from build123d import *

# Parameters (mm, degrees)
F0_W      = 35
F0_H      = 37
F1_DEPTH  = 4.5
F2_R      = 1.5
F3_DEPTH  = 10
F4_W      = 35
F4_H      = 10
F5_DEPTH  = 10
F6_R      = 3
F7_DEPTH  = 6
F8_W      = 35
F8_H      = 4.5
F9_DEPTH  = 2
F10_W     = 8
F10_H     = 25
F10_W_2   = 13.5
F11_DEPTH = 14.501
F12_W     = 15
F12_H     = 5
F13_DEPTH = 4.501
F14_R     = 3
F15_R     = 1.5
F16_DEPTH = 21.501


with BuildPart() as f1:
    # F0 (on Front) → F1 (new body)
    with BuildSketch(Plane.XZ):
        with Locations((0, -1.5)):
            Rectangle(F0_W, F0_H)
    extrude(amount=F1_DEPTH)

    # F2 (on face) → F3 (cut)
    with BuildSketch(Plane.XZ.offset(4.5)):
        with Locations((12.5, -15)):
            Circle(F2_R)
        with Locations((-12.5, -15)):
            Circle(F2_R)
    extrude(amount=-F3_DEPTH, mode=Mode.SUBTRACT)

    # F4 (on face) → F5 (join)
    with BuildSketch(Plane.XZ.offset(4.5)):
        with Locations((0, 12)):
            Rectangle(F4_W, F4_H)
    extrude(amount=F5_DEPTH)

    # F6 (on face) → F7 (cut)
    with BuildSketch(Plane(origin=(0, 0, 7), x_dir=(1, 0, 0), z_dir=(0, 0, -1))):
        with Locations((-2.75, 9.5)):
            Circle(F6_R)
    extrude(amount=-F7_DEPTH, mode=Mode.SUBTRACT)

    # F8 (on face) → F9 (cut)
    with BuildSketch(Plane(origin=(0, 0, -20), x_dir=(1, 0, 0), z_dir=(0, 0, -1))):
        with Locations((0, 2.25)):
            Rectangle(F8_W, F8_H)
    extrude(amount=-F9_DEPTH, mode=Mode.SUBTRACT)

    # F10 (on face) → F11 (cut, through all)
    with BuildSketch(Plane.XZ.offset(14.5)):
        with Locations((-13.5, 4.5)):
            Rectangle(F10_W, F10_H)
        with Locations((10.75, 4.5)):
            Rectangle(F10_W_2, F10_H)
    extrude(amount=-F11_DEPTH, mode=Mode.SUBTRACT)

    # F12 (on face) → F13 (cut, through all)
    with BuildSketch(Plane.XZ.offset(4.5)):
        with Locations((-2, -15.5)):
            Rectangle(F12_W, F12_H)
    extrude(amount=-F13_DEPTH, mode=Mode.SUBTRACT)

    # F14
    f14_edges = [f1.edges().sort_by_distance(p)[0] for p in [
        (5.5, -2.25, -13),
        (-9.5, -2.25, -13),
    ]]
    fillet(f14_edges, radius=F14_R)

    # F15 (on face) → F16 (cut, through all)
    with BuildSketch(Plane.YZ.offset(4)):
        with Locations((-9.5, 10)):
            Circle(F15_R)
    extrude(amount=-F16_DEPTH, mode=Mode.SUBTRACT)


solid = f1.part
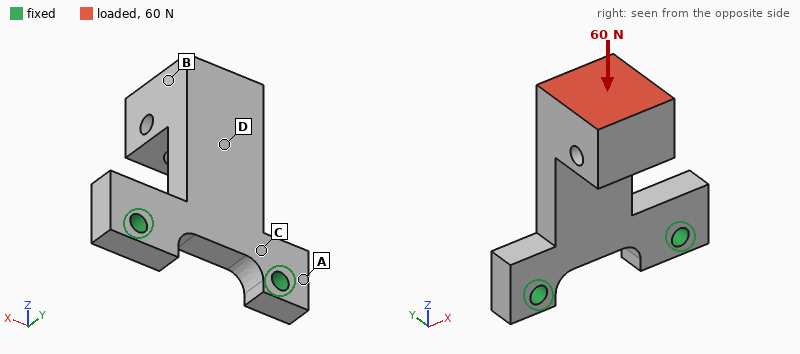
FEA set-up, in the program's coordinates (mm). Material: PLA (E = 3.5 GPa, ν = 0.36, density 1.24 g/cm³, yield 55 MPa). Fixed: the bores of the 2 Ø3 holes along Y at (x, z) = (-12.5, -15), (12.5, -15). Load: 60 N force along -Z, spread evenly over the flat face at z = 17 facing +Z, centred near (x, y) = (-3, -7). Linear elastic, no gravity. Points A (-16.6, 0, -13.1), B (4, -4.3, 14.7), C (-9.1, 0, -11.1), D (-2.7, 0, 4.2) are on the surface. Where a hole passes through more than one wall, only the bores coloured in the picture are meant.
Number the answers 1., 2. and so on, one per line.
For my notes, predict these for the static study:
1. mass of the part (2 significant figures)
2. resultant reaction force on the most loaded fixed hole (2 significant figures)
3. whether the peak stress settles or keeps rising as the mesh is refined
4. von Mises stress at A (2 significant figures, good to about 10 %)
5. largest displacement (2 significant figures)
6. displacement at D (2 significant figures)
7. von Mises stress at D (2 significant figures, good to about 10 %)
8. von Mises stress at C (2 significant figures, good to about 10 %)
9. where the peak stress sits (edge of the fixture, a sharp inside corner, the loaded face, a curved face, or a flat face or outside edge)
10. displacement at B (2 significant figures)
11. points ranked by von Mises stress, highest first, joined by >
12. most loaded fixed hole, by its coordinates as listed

1. 4.8 g
2. 42 N
3. keeps rising
4. 2.0 MPa
5. 0.58 mm
6. 0.21 mm
7. 5.2 MPa
8. 8.0 MPa
9. edge of the fixture
10. 0.45 mm
11. C > D > A > B
12. (-12.5, -15)
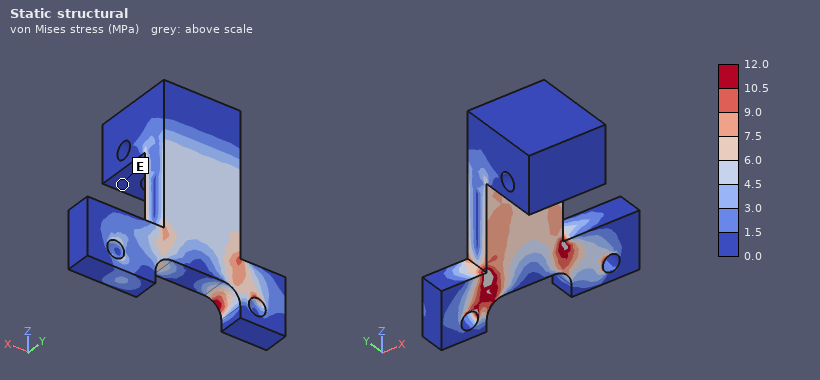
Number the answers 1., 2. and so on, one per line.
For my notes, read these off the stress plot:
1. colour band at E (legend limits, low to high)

1. 0.0 to 1.5 MPa
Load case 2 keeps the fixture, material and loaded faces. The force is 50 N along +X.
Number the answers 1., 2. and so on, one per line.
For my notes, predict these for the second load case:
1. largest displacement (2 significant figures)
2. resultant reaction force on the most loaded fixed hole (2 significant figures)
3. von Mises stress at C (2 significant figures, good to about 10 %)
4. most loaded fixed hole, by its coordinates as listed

1. 0.32 mm
2. 91 N
3. 7.9 MPa
4. (12.5, -15)
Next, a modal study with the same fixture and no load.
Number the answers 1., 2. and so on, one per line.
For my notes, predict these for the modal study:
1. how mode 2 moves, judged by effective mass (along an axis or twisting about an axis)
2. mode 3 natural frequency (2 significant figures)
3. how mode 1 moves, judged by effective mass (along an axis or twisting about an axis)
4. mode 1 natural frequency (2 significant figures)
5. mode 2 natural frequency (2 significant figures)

1. along X
2. 3100 Hz
3. along Y
4. 620 Hz
5. 1700 Hz
